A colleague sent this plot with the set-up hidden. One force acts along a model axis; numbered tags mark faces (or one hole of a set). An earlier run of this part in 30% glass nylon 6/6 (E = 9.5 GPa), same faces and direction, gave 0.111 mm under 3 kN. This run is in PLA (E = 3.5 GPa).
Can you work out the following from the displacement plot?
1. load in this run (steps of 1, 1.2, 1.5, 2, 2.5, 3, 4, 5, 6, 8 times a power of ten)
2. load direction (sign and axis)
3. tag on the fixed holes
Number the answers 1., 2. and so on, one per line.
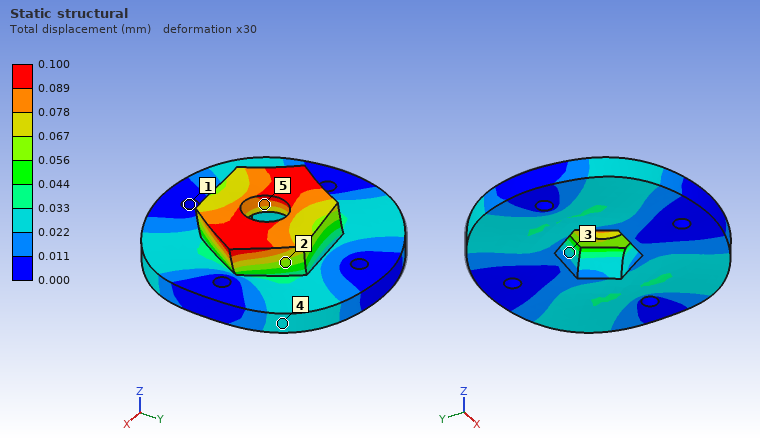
1. 1 kN
2. +X
3. 1
